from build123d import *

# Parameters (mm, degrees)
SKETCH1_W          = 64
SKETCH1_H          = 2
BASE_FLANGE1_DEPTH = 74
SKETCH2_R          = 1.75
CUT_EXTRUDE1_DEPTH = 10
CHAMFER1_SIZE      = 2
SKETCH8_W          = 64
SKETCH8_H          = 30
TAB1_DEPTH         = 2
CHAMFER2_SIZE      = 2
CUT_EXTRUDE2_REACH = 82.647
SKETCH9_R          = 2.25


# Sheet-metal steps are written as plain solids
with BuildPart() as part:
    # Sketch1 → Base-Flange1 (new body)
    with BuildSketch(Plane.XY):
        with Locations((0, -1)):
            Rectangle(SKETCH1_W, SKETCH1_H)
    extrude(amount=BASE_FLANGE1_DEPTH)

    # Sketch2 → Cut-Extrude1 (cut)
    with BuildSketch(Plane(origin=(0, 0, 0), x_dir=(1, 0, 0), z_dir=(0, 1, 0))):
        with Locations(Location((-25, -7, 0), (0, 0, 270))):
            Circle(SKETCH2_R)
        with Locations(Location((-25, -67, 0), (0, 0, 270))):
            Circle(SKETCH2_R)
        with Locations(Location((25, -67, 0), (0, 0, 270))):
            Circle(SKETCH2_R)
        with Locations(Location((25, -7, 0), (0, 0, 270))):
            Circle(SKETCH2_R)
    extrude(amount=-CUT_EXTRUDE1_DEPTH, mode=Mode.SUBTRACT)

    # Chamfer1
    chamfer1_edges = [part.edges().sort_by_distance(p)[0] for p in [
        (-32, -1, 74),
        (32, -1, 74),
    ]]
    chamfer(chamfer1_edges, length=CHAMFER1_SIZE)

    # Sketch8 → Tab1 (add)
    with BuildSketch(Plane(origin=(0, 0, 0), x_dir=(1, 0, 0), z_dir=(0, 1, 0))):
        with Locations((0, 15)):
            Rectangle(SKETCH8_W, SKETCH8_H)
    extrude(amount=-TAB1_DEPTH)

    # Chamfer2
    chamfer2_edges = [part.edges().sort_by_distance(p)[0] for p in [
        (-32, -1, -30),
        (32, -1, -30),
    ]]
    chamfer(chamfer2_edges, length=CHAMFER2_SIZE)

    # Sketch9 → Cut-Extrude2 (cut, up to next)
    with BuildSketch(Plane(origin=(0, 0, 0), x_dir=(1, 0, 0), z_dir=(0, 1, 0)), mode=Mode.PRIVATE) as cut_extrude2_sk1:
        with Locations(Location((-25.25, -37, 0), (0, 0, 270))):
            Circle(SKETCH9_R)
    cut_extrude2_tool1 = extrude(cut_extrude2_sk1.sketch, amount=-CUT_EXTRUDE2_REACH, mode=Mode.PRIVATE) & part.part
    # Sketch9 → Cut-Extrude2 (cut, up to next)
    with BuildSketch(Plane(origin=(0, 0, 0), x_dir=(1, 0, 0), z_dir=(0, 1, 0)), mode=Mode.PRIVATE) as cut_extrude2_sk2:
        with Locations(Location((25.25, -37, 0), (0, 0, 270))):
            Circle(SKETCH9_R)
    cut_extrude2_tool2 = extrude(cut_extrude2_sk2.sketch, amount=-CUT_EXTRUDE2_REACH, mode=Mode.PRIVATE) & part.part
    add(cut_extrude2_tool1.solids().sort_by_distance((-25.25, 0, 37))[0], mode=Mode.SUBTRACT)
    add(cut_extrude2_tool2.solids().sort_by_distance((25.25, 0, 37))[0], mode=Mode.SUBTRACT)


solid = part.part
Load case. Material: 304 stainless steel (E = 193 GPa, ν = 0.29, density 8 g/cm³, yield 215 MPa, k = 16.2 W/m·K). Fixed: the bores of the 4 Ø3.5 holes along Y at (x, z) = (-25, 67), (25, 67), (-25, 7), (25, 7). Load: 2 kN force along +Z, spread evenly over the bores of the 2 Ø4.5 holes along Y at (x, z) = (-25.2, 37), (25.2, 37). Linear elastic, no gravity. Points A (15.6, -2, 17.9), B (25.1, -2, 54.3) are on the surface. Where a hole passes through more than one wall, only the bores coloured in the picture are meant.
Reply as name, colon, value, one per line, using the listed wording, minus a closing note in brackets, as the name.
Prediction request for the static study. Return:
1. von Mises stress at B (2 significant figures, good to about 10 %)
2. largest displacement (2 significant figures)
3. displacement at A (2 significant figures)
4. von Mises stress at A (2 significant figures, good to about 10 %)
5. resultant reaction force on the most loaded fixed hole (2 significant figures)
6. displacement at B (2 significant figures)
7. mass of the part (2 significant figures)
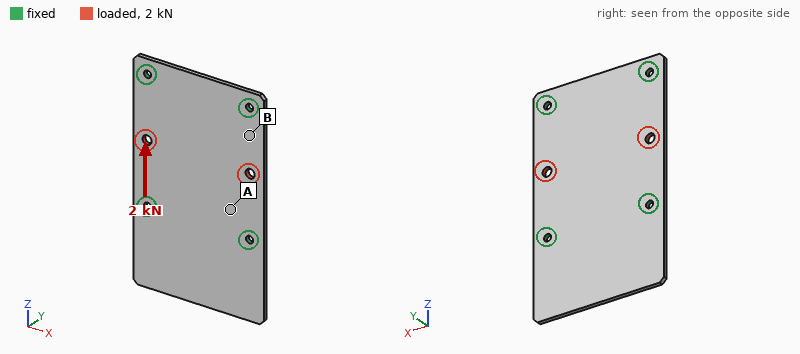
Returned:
von Mises stress at B: 15 MPa
largest displacement: 3.0 µm
displacement at A: 1.0 µm
von Mises stress at A: 6.0 MPa
resultant reaction force on the most loaded fixed hole: 530 N
displacement at B: 1.2 µm
mass of the part: 110 g
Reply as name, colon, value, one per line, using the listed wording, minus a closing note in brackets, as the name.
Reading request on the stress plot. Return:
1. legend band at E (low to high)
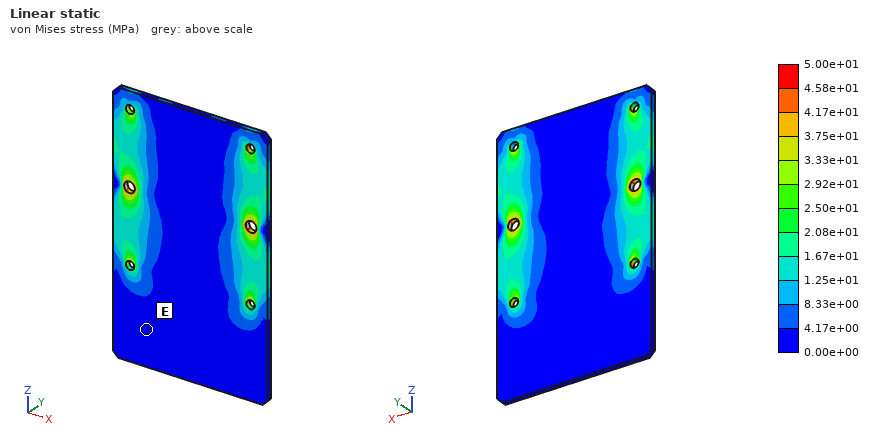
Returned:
legend band at E: 0.00e+00 to 4.17e+00 MPa
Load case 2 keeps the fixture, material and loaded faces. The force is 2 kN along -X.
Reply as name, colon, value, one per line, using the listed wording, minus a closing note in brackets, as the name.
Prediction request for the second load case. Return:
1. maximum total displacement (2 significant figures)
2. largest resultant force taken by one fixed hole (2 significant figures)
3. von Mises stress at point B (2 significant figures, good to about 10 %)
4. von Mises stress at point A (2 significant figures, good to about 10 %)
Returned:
maximum total displacement: 6.2 µm
largest resultant force taken by one fixed hole: 560 N
von Mises stress at point B: 8.6 MPa
von Mises stress at point A: 18 MPa
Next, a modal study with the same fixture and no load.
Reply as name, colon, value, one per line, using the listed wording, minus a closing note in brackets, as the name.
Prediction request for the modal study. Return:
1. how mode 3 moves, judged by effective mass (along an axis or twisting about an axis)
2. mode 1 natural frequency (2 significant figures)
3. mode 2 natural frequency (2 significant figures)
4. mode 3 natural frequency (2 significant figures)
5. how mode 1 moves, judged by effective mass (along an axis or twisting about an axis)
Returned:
how mode 3 moves, judged by effective mass: along Y
mode 1 natural frequency: 1000 Hz
mode 2 natural frequency: 2000 Hz
mode 3 natural frequency: 2300 Hz
how mode 1 moves, judged by effective mass: along Y
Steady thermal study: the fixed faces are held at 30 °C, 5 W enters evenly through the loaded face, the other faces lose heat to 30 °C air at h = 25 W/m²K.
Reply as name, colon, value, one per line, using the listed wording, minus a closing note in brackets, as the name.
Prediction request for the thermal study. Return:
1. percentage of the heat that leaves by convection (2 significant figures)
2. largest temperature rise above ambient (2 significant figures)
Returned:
percentage of the heat that leaves by convection: 59 %
largest temperature rise above ambient: 46 K
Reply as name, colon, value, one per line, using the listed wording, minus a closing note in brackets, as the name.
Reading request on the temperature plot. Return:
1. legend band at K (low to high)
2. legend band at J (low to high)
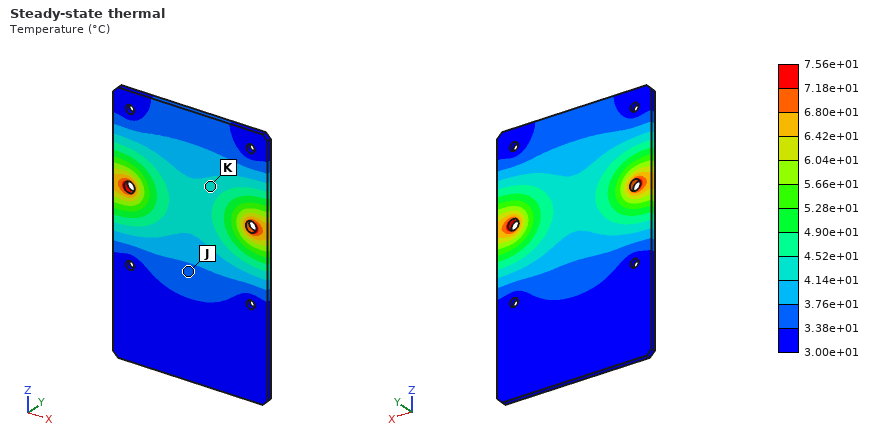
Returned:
legend band at K: 4.14e+01 to 4.52e+01 °C
legend band at J: 3.38e+01 to 3.76e+01 °C
